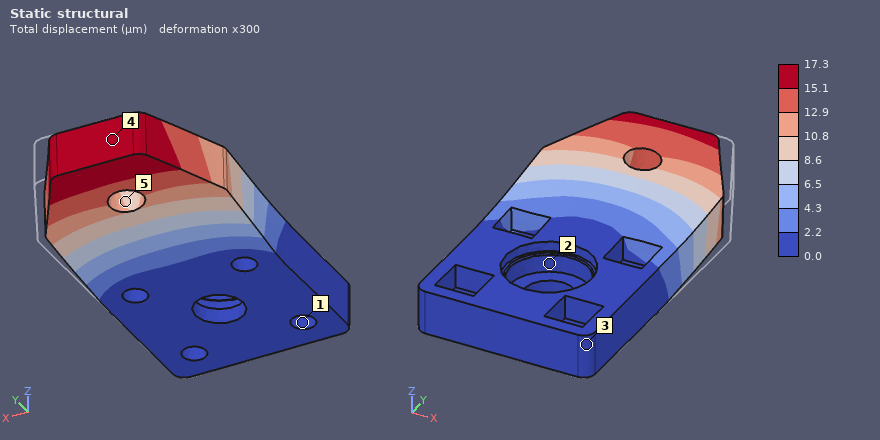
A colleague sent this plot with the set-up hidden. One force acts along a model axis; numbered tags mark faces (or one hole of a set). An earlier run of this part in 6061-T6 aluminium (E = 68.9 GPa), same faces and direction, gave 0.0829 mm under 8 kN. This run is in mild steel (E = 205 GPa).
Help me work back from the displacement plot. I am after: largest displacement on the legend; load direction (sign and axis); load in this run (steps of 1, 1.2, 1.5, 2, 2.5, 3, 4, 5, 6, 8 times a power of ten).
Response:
17.3 µm
-X
5 kN
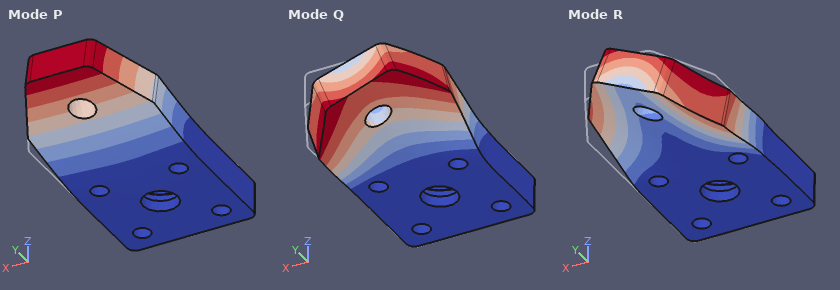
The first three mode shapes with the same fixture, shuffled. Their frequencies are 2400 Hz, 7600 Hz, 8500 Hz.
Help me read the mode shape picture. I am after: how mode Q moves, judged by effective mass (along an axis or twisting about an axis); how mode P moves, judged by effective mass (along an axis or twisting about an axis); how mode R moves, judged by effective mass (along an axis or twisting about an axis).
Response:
along X
along Z
along X
